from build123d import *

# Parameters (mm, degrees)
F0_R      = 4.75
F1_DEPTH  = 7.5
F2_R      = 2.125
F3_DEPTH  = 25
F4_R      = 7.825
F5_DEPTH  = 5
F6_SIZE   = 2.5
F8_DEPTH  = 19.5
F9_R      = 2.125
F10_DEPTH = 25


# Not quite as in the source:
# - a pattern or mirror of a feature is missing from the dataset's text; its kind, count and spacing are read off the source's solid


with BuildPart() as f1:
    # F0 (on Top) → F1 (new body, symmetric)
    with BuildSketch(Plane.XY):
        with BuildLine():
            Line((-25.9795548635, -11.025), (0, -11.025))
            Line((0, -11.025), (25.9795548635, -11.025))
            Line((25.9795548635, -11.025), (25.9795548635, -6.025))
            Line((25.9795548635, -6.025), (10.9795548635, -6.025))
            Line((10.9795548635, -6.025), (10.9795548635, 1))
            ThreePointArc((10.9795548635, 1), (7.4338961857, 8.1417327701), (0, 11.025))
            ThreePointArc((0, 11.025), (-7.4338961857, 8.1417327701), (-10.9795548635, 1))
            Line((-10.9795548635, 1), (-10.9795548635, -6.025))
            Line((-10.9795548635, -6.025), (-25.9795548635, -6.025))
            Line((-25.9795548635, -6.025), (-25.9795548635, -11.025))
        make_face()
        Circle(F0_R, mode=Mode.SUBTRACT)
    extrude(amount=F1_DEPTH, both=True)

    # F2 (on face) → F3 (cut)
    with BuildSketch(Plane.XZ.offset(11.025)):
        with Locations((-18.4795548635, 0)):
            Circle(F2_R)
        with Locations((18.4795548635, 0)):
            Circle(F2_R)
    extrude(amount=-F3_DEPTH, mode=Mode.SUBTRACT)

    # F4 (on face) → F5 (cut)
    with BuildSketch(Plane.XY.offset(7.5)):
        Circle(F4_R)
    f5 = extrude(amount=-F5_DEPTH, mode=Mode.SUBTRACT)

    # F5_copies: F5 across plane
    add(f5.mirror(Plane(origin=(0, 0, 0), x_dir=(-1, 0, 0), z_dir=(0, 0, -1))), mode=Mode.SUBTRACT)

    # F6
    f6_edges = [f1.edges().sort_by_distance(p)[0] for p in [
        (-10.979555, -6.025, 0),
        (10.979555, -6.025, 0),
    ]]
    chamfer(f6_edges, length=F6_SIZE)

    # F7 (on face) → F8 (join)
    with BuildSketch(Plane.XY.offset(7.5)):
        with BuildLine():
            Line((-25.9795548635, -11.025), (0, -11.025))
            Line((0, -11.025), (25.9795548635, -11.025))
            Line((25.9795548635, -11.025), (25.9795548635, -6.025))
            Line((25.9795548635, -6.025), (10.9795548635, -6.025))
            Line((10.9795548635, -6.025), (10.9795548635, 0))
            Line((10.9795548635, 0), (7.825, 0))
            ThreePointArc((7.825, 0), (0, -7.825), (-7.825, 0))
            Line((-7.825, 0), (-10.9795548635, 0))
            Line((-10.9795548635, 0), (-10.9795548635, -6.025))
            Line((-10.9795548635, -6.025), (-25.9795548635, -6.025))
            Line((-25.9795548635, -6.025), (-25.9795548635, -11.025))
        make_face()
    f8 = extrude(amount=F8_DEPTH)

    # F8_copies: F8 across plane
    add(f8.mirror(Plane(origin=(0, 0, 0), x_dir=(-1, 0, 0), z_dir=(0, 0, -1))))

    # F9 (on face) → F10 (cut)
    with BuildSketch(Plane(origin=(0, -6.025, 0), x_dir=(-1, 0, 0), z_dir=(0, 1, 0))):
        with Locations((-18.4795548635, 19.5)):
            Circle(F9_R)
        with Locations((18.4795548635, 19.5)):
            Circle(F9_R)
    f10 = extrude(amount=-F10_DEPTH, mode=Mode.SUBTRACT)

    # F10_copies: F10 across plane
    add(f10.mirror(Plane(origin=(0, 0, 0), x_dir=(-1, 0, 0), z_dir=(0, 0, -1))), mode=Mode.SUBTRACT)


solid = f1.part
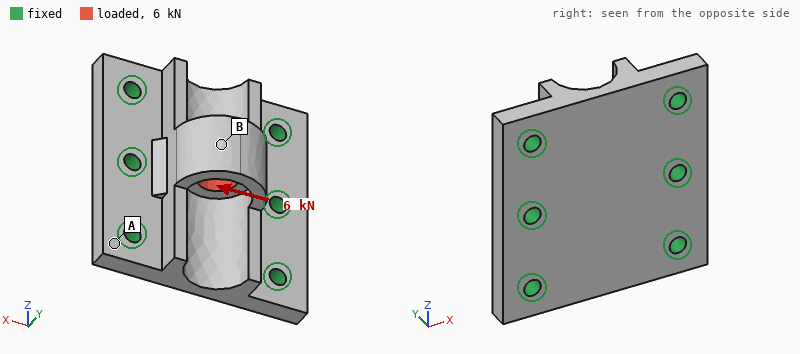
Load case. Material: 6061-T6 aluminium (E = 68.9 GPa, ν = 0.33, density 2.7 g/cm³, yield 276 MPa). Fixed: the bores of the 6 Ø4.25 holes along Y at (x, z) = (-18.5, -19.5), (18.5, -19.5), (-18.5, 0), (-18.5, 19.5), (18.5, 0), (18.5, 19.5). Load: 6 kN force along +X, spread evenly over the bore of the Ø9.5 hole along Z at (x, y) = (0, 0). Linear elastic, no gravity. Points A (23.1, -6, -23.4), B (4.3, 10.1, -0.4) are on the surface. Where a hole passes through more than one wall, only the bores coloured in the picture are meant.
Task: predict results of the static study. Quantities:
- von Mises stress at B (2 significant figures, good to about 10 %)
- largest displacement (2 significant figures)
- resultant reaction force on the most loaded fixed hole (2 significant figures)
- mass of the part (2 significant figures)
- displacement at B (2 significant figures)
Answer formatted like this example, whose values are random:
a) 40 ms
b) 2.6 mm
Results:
a) 32 MPa
b) 39 µm
c) 2.4 kN
d) 48 g
e) 36 µm
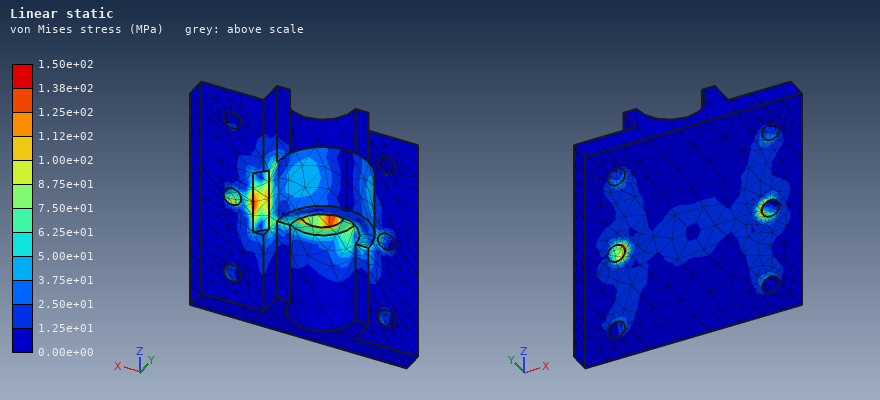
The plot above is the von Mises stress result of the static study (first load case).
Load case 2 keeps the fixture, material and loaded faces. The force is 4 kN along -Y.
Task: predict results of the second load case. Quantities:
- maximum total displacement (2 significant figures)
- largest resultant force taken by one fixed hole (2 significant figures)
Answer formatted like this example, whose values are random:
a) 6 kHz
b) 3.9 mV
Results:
a) 23 µm
b) 1.4 kN
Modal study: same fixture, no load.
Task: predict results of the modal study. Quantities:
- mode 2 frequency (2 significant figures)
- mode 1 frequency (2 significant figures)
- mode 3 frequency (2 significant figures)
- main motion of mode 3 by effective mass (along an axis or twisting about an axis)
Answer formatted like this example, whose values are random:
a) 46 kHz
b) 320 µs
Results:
a) 16 kHz
b) 16 kHz
c) 22 kHz
d) along X
